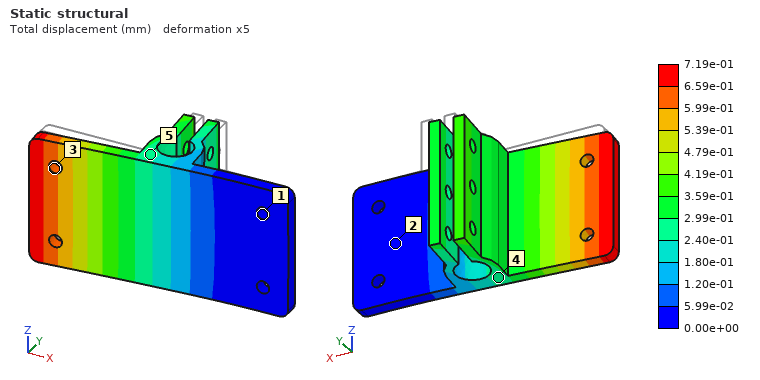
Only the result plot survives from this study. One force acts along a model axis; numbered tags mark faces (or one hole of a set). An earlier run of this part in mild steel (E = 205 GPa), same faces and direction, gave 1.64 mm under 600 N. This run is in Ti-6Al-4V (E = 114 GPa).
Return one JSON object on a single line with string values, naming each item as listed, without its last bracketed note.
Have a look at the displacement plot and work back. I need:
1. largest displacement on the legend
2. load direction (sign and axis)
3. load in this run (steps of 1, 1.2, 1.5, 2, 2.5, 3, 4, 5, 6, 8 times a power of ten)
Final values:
{"largest displacement on the legend": "7.19e-01 mm", "load direction": "-Y", "load in this run": "150 N"}
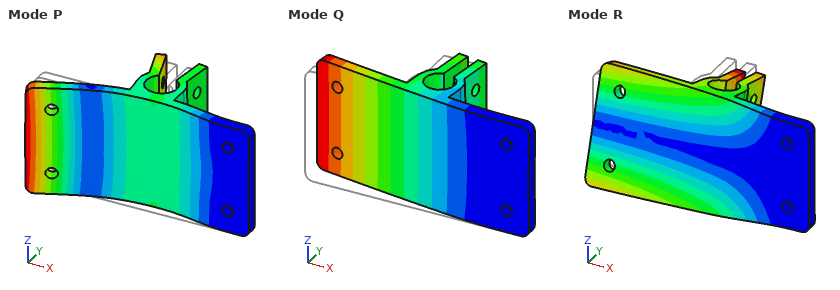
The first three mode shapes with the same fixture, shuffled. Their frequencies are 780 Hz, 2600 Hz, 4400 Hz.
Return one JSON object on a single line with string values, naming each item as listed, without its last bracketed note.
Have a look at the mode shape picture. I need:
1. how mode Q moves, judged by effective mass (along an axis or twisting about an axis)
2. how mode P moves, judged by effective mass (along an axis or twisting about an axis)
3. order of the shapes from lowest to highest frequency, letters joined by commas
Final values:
{"how mode Q moves, judged by effective mass": "along Y", "how mode P moves, judged by effective mass": "along Y", "order of the shapes from lowest to highest frequency, letters joined by commas": "Q, R, P"}
